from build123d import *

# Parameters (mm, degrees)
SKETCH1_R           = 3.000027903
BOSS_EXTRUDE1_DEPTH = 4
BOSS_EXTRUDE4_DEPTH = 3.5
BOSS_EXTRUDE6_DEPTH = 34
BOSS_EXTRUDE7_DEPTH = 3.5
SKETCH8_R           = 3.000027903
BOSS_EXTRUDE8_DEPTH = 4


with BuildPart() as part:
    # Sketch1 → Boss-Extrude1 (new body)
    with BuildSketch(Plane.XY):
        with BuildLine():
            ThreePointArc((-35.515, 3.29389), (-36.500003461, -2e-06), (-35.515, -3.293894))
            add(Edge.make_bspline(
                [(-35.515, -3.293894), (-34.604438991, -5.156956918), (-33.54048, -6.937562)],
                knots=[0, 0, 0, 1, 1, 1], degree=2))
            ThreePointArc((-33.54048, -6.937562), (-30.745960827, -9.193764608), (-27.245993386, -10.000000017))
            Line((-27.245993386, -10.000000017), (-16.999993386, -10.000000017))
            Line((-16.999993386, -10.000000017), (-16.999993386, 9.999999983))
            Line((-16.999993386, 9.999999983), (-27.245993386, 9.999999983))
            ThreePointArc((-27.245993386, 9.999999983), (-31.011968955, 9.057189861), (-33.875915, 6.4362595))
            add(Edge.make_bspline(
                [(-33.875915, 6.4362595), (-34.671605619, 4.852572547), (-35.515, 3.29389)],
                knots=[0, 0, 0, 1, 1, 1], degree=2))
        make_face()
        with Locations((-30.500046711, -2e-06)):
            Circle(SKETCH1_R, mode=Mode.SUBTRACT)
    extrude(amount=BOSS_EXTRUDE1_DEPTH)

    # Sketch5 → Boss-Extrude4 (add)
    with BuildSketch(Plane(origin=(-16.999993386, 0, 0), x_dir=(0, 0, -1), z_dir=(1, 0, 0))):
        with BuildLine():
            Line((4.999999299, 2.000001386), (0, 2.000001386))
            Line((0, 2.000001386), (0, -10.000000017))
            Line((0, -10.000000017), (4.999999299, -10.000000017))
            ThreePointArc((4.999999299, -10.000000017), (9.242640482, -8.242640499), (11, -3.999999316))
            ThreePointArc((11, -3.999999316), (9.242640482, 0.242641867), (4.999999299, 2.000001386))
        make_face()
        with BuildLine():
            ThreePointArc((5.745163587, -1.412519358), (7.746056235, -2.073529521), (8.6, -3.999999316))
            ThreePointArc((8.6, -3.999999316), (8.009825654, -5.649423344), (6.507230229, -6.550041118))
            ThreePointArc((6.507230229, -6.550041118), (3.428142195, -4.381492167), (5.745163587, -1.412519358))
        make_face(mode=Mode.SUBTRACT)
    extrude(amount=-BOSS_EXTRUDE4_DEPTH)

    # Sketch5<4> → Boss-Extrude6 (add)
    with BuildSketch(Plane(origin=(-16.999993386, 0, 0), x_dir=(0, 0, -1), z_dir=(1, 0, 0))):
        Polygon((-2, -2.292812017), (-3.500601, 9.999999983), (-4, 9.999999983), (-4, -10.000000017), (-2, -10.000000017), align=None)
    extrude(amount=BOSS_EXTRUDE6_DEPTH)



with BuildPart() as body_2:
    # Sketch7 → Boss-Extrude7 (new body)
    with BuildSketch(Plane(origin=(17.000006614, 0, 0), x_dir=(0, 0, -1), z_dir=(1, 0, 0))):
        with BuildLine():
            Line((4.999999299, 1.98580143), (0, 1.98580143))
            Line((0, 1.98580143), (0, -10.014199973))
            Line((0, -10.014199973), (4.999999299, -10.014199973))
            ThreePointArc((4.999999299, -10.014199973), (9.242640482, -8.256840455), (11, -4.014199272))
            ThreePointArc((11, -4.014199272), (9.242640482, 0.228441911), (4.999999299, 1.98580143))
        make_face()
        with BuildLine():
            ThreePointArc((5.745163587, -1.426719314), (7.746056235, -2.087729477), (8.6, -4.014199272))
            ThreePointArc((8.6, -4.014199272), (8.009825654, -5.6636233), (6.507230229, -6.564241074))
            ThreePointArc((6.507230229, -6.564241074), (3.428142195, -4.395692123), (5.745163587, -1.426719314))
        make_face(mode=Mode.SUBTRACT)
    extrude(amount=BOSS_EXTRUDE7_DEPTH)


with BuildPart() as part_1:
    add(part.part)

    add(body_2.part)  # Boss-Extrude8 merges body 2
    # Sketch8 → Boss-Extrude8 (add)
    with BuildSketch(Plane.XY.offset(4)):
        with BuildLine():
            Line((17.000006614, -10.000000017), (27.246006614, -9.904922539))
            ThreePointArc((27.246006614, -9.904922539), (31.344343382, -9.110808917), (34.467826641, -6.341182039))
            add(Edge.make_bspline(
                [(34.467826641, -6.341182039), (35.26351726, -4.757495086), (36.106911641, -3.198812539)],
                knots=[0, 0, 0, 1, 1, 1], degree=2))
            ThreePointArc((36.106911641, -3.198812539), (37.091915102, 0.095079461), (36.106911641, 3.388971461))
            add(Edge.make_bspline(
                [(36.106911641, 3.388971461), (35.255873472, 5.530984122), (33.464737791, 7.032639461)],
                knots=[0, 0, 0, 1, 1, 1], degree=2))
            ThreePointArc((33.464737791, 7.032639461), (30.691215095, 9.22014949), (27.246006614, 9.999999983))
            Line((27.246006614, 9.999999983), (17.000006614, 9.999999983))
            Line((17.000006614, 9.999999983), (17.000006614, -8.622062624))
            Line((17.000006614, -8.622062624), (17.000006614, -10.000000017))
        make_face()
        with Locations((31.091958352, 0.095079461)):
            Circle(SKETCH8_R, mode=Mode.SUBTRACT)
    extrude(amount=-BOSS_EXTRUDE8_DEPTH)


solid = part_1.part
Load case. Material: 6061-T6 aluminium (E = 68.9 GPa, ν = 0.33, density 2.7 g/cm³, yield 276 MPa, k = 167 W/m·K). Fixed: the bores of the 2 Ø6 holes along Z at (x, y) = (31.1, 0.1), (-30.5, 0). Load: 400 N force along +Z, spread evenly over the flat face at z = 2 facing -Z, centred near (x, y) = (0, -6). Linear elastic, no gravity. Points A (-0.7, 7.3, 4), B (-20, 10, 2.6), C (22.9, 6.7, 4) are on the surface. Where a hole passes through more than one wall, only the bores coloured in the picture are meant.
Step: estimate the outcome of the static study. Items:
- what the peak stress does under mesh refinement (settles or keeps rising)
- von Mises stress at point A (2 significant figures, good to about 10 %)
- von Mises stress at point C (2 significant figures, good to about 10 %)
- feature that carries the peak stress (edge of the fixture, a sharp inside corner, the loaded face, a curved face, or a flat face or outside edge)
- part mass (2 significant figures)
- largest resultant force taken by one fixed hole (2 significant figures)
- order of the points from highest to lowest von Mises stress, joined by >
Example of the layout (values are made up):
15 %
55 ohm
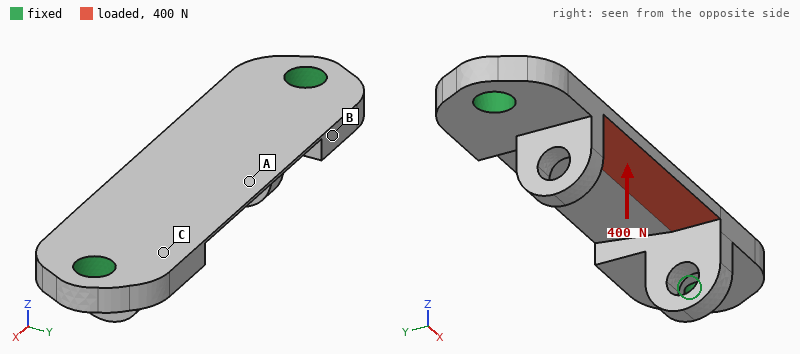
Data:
keeps rising
45 MPa
27 MPa
edge of the fixture
12 g
380 N
A > C > B
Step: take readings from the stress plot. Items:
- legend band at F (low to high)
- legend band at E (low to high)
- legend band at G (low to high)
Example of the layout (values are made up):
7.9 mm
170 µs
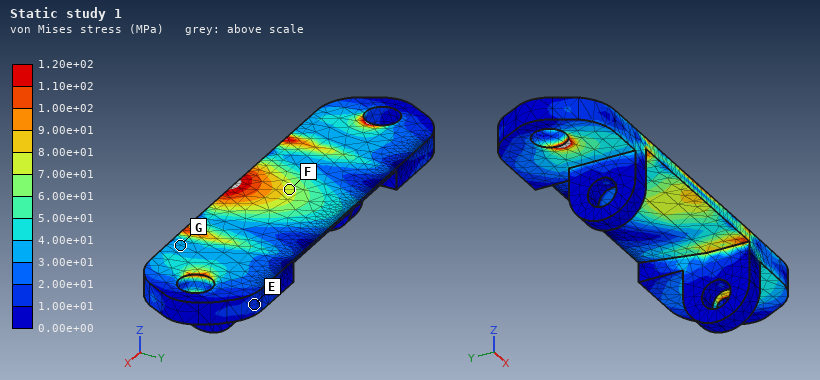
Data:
7.00e+01 to 8.00e+01 MPa
1.00e+01 to 2.00e+01 MPa
3.00e+01 to 4.00e+01 MPa
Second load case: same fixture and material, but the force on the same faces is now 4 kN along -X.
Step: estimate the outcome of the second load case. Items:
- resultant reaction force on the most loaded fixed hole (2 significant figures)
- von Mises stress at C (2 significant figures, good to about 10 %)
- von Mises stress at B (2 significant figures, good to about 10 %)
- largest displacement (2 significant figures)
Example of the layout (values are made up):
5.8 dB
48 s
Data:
2.1 kN
44 MPa
11 MPa
56 µm
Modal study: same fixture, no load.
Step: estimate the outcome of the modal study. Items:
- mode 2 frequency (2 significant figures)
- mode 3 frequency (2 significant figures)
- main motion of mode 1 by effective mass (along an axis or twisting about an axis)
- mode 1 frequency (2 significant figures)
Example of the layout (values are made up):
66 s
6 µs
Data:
8600 Hz
9500 Hz
along Z
5300 Hz
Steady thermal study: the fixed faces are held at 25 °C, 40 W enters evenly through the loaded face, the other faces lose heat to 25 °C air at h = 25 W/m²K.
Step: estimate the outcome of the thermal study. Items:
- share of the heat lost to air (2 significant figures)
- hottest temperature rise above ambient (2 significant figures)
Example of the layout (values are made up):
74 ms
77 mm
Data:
4.6 %
62 K
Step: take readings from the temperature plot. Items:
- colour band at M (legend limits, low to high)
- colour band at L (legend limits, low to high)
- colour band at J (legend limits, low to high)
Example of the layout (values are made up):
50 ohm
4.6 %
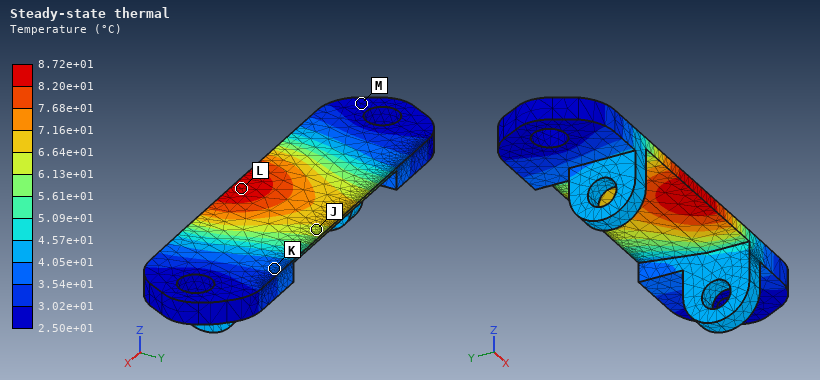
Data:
2.50e+01 to 3.02e+01 °C
8.20e+01 to 8.72e+01 °C
6.13e+01 to 6.64e+01 °C
